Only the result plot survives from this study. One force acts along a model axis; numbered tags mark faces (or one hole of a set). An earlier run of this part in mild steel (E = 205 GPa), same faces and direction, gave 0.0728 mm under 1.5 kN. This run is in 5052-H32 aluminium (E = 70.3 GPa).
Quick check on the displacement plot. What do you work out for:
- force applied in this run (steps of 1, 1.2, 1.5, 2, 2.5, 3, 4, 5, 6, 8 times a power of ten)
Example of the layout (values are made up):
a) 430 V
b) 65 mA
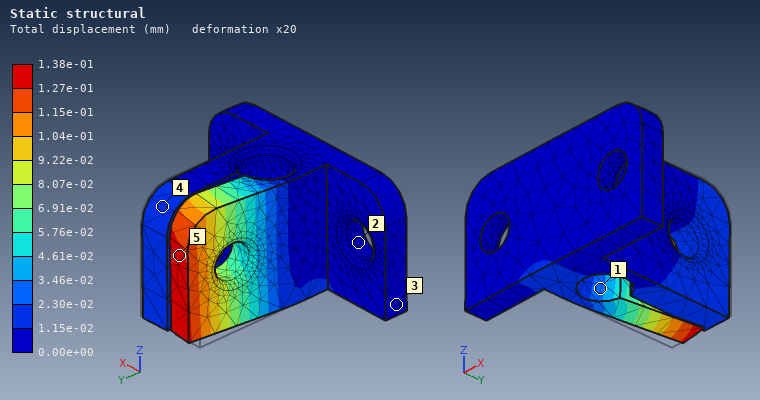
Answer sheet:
a) 1 kN
